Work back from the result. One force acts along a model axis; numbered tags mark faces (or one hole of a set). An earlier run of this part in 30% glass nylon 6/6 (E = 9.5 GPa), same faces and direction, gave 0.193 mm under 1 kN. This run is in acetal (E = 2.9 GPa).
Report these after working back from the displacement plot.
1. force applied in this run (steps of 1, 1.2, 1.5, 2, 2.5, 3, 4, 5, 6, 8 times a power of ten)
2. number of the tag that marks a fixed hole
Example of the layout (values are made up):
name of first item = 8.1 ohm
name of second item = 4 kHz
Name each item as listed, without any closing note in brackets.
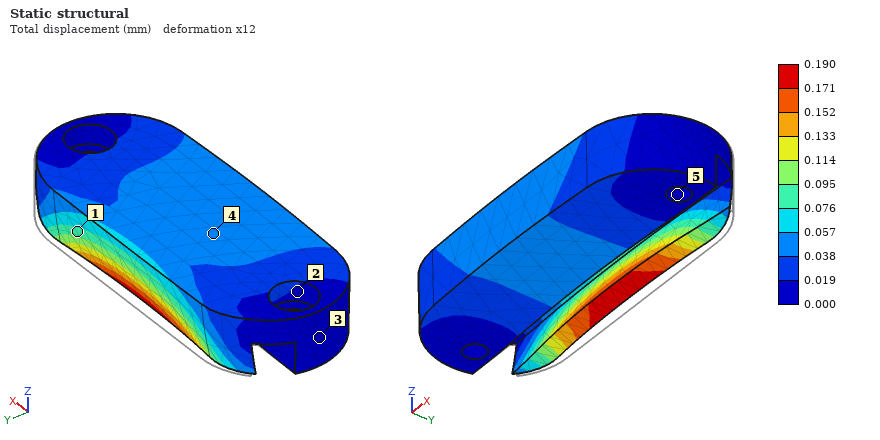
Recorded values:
force applied in this run = 300 N
number of the tag that marks a fixed hole = 5
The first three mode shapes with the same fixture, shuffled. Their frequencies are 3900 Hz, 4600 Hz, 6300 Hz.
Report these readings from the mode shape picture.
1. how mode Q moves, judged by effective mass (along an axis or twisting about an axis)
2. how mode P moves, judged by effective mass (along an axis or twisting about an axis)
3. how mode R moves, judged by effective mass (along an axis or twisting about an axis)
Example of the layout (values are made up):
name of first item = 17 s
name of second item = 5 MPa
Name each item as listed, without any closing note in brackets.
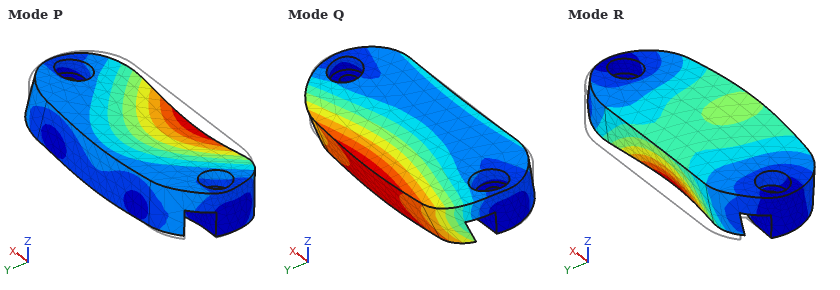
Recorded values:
how mode Q moves, judged by effective mass = along Z
how mode P moves, judged by effective mass = along Z
how mode R moves, judged by effective mass = along Y
